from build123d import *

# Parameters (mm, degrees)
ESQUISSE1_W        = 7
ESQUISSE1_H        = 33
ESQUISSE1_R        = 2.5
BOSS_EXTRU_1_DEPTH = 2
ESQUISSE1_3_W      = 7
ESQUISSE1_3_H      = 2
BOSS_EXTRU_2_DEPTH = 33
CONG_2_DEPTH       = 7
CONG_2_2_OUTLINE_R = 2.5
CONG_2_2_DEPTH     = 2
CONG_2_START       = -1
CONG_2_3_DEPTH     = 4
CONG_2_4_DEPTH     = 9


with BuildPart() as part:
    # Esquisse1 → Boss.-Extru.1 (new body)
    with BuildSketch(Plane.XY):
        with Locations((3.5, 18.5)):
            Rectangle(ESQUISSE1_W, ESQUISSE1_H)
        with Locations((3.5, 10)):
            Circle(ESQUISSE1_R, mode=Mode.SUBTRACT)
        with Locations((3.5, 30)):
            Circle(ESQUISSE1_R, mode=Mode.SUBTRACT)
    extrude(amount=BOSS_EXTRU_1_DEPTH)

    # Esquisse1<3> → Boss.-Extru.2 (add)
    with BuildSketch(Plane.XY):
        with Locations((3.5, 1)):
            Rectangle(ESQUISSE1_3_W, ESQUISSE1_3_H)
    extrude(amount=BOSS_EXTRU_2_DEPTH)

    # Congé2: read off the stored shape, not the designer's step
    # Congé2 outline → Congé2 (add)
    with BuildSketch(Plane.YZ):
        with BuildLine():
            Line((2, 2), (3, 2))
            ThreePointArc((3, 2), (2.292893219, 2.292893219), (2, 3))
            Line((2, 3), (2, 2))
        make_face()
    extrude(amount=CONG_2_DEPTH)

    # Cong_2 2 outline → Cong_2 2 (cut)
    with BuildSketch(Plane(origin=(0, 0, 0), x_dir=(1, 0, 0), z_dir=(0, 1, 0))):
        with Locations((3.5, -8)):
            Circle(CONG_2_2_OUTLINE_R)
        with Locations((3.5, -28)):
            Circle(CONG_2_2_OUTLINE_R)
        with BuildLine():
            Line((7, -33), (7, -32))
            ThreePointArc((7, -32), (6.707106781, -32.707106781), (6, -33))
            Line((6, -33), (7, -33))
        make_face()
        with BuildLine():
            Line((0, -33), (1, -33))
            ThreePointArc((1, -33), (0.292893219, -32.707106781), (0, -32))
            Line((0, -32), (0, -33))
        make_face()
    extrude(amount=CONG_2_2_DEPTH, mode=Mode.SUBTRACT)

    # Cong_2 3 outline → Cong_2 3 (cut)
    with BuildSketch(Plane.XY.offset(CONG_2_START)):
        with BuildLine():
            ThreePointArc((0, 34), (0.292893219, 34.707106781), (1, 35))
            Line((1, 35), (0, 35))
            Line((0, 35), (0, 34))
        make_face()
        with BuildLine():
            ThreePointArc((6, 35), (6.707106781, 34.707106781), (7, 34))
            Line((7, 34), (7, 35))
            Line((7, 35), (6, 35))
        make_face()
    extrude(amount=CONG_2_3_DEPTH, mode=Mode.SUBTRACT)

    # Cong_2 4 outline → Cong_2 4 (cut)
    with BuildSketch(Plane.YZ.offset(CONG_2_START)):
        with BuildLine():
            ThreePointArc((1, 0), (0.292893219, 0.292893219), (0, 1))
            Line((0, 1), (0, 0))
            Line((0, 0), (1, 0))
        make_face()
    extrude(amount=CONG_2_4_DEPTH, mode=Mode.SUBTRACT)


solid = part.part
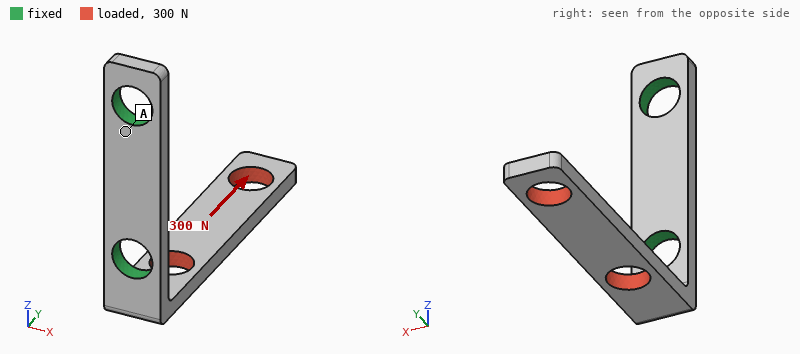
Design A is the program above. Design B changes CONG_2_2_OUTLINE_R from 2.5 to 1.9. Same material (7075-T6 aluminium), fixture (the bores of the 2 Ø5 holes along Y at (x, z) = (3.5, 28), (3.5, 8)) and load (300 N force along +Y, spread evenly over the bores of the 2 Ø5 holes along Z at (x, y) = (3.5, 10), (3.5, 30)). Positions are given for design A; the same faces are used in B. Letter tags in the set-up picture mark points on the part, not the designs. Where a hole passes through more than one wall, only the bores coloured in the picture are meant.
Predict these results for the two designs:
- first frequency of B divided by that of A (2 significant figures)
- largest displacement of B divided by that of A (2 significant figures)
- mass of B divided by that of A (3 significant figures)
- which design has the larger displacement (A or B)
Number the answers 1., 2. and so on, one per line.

1. 0.98
2. 1.3
3. 1.04
4. B
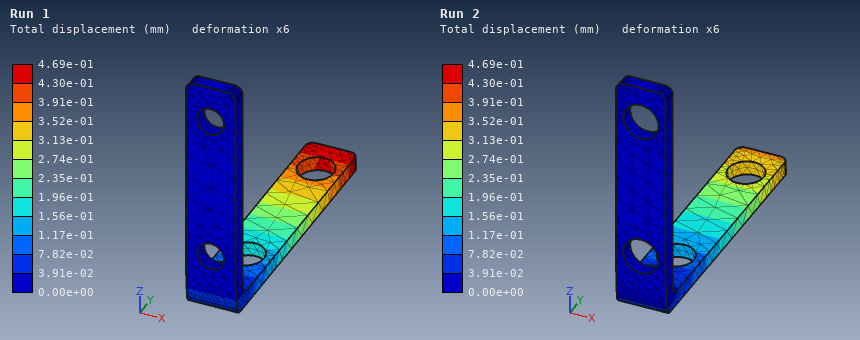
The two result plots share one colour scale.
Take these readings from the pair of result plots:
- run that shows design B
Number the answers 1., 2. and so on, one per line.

1. Run 1
